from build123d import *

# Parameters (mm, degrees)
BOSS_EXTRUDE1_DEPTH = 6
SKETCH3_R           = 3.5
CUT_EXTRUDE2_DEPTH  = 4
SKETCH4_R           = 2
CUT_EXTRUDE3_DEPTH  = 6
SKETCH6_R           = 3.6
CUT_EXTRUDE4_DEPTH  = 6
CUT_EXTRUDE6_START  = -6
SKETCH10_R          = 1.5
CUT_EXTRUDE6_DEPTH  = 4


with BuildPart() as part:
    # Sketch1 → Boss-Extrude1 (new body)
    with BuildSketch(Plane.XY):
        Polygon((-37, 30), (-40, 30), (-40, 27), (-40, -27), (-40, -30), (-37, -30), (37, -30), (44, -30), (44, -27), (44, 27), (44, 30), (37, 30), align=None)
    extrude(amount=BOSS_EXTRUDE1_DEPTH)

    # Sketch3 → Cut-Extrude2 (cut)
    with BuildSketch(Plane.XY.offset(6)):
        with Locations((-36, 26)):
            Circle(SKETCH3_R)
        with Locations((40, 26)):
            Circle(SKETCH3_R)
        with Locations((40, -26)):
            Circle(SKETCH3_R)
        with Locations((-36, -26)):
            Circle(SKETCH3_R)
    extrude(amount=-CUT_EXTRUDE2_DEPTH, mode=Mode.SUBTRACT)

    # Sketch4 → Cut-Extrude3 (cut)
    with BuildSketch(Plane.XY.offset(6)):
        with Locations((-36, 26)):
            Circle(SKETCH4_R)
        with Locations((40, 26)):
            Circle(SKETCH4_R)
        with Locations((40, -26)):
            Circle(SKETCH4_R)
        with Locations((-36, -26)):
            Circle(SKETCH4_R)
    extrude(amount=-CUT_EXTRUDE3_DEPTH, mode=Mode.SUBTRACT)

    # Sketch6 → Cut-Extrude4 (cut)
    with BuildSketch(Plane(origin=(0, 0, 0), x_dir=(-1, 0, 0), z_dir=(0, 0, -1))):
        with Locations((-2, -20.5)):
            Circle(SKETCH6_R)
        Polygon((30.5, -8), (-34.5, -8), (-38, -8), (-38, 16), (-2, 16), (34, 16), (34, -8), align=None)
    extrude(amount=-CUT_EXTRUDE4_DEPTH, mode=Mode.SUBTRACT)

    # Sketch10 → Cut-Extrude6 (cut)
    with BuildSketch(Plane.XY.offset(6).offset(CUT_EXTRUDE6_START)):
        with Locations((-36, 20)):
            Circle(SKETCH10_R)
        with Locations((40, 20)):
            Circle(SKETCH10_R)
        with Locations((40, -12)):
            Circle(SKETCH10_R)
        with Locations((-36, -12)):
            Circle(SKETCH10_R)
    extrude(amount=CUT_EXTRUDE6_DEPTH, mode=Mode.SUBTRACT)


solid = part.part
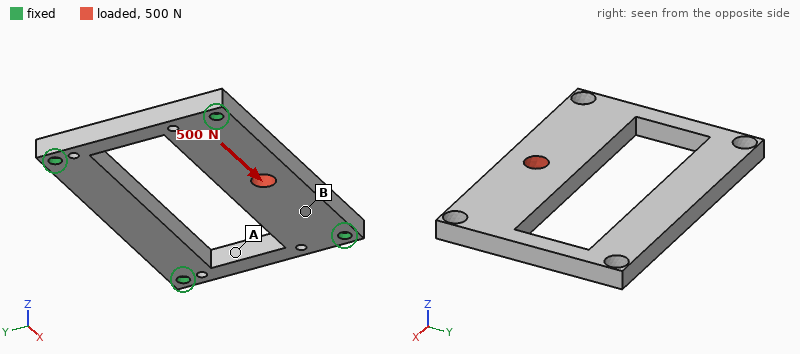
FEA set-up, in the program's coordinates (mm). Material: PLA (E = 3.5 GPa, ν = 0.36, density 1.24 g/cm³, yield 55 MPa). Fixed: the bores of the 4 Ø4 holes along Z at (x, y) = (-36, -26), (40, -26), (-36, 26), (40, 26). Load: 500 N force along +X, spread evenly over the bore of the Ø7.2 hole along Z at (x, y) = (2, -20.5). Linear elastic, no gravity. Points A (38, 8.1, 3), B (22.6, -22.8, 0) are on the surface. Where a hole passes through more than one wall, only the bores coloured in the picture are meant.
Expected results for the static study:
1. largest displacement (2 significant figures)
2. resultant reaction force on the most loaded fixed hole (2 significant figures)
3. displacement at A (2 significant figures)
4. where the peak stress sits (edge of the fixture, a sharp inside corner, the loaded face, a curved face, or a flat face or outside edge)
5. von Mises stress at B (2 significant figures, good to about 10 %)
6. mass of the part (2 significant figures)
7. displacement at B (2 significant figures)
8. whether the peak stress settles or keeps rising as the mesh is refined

52 µm
250 N
16 µm
edge of the fixture
4.2 MPa
23 g
40 µm
keeps rising
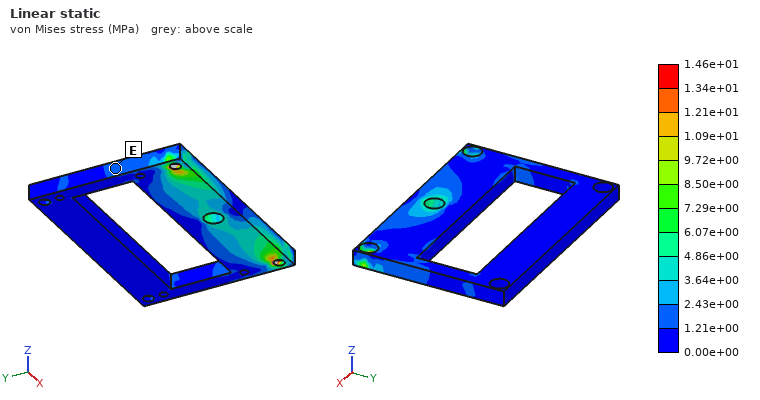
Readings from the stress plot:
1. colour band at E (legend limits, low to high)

1.21e+00 to 2.43e+00 MPa
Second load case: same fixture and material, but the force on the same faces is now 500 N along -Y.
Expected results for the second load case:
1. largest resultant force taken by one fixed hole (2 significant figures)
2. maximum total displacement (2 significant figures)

300 N
0.28 mm
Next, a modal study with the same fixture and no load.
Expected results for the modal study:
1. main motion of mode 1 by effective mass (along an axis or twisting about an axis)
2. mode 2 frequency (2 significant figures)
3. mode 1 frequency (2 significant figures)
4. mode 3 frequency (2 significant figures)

along Z
1300 Hz
1100 Hz
2300 Hz
